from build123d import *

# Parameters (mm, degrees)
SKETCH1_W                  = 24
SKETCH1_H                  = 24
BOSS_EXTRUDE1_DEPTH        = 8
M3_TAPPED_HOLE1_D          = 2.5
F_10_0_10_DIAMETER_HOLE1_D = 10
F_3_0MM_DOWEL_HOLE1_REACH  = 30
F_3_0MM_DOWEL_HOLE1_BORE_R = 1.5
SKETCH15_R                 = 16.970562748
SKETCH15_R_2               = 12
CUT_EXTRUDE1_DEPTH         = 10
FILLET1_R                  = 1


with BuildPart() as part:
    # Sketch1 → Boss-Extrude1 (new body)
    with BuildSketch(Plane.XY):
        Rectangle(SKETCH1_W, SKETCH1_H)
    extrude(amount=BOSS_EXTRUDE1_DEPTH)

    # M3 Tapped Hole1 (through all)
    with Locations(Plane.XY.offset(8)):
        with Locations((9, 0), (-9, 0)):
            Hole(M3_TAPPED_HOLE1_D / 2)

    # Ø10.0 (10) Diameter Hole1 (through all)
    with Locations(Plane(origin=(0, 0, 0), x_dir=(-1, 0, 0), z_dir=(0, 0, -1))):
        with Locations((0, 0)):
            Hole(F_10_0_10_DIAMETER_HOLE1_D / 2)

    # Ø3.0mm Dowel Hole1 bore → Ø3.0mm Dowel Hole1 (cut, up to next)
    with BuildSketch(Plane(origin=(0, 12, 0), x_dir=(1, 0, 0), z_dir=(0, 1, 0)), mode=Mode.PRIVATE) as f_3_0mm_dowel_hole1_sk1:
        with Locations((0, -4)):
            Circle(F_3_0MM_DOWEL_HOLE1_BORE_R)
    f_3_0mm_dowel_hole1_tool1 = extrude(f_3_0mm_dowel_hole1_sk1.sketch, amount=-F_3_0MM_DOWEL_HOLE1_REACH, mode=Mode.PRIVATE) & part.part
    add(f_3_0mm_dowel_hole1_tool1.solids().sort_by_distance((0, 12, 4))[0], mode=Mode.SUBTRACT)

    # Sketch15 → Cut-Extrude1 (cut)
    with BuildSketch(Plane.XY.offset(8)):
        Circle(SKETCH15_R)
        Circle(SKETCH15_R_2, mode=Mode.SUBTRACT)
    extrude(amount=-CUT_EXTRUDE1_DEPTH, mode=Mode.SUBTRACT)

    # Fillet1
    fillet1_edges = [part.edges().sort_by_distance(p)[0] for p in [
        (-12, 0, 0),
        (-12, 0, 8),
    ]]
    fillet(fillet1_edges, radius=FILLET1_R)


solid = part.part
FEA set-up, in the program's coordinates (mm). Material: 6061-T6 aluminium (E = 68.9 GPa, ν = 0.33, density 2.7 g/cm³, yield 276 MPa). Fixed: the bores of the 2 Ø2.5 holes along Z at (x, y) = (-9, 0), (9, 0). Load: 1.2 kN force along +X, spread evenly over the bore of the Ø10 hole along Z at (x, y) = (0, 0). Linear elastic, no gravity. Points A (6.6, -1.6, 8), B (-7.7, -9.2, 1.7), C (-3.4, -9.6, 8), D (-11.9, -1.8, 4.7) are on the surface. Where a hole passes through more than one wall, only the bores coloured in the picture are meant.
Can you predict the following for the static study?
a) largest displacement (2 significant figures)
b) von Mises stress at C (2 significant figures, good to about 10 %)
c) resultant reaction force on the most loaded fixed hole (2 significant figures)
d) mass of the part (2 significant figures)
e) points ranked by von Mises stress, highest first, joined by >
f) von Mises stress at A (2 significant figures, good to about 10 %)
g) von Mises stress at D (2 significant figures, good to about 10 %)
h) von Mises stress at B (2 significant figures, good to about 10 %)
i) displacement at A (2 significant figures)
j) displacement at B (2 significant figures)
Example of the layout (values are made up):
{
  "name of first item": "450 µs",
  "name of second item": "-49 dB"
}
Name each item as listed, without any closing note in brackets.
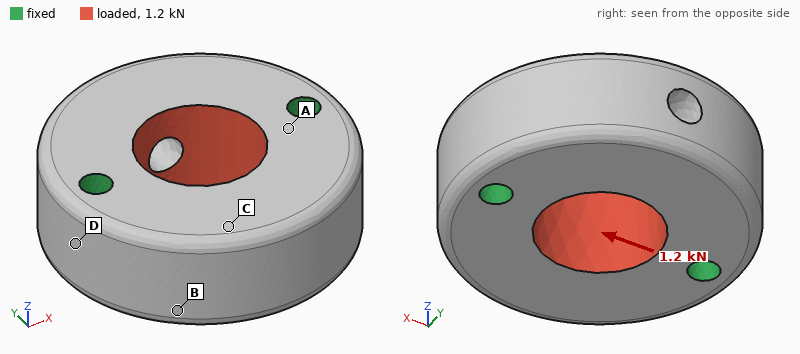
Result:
{
  "largest displacement": "1.5 µm",
  "von Mises stress at C": "2.0 MPa",
  "resultant reaction force on the most loaded fixed hole": "600 N",
  "mass of the part": "7.6 g",
  "points ranked by von Mises stress, highest first, joined by >": "A > D > B > C",
  "von Mises stress at A": "12 MPa",
  "von Mises stress at D": "6.8 MPa",
  "von Mises stress at B": "3.3 MPa",
  "displacement at A": "0.43 µm",
  "displacement at B": "1.2 µm"
}
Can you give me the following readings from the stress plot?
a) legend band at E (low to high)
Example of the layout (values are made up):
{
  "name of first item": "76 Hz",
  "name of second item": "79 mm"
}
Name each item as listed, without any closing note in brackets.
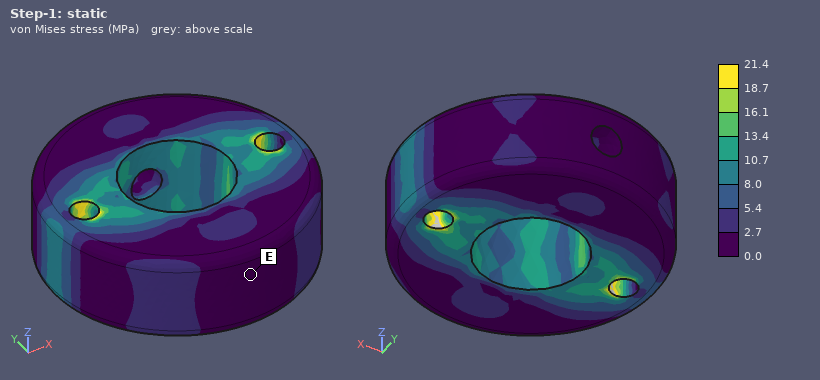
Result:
{
  "legend band at E": "0.0 to 2.7 MPa"
}
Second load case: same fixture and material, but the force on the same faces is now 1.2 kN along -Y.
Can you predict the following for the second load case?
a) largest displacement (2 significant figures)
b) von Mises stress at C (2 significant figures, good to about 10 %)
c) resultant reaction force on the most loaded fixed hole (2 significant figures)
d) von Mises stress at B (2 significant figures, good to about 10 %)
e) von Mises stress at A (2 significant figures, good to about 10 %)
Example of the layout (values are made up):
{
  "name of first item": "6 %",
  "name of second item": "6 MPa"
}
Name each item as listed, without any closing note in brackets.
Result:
{
  "largest displacement": "1.5 µm",
  "von Mises stress at C": "4.8 MPa",
  "resultant reaction force on the most loaded fixed hole": "600 N",
  "von Mises stress at B": "3.9 MPa",
  "von Mises stress at A": "11 MPa"
}
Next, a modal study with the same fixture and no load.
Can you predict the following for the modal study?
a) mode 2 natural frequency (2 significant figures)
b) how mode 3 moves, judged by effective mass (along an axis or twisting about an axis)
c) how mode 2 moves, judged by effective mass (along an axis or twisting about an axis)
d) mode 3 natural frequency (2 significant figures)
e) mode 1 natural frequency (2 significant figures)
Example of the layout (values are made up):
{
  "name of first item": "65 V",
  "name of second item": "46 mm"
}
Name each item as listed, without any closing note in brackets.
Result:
{
  "mode 2 natural frequency": "36 kHz",
  "how mode 3 moves, judged by effective mass": "twisting about Z",
  "how mode 2 moves, judged by effective mass": "along Z",
  "mode 3 natural frequency": "50 kHz",
  "mode 1 natural frequency": "32 kHz"
}
